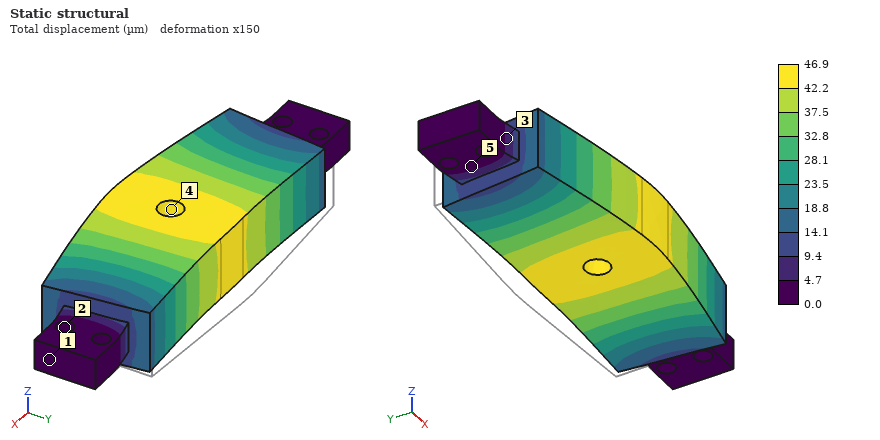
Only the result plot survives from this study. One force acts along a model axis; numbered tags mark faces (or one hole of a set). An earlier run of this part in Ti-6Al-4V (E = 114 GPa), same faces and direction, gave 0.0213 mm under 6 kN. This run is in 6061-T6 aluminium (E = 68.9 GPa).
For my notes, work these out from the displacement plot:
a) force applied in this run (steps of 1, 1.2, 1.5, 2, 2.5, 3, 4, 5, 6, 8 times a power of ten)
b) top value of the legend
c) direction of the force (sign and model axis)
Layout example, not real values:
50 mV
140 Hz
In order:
8 kN
46.9 µm
-Y
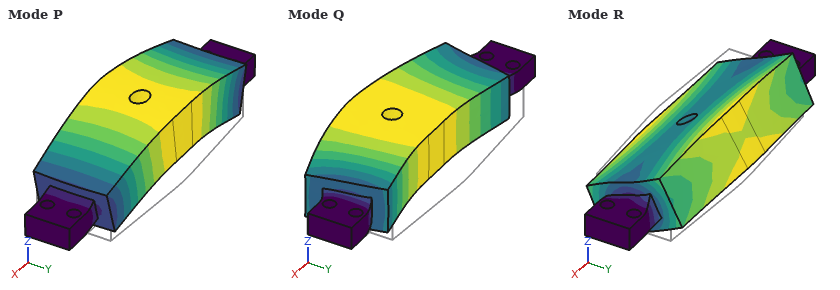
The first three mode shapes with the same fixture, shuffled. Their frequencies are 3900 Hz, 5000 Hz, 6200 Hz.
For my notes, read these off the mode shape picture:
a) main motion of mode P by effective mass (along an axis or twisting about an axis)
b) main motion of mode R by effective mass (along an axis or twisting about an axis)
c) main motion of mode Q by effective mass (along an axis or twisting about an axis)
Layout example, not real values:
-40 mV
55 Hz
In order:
along Z
twisting about X
along Y
